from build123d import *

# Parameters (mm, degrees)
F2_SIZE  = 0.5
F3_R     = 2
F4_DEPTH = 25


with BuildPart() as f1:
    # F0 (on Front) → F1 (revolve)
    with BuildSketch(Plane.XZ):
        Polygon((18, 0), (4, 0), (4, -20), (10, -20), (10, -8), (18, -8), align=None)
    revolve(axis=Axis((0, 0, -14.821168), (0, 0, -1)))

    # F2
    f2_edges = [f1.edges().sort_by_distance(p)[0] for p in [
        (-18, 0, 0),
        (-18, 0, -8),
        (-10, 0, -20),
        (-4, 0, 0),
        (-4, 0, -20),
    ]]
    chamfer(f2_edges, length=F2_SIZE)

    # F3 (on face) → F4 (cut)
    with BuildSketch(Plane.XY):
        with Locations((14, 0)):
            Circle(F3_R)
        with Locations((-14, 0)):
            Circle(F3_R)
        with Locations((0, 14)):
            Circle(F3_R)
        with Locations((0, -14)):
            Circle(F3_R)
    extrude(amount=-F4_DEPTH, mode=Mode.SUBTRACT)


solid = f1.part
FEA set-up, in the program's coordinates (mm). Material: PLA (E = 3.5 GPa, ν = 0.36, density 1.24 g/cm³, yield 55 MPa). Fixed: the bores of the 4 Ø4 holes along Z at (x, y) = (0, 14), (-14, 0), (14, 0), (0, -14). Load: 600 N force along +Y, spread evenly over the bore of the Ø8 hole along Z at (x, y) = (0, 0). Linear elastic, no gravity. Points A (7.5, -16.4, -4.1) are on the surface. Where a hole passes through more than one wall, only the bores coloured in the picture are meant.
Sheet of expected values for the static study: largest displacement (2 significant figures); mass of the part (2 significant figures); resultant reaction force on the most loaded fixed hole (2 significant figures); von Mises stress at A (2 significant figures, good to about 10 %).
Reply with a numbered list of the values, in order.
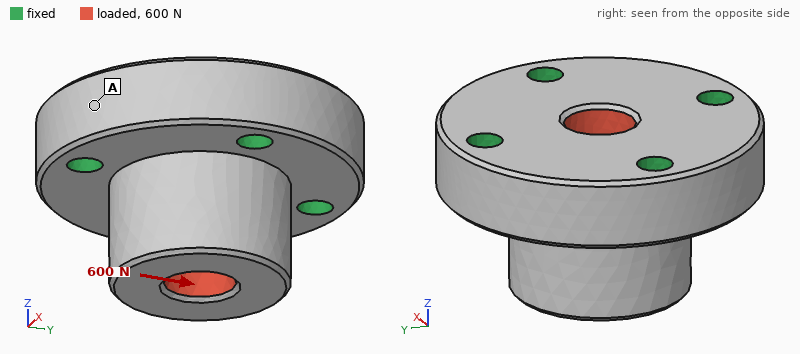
1. 26 µm
2. 13 g
3. 230 N
4. 0.99 MPa
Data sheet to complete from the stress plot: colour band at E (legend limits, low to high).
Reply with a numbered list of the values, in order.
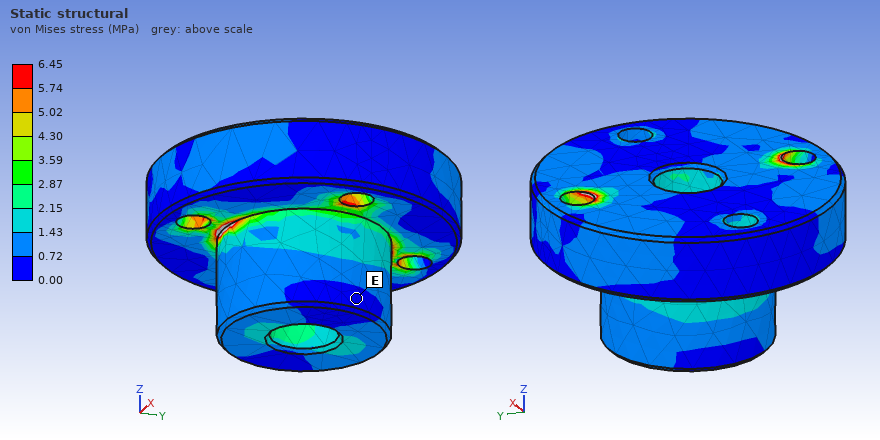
1. 0.00 to 0.72 MPa
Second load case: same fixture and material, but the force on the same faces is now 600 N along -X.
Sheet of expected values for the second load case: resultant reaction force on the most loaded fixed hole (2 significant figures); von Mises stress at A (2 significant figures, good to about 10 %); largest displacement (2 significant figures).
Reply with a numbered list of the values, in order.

1. 230 N
2. 0.66 MPa
3. 26 µm
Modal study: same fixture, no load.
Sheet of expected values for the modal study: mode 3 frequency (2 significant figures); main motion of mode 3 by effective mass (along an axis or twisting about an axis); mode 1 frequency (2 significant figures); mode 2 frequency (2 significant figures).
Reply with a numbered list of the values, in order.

1. 14 kHz
2. along Z
3. 11 kHz
4. 11 kHz
